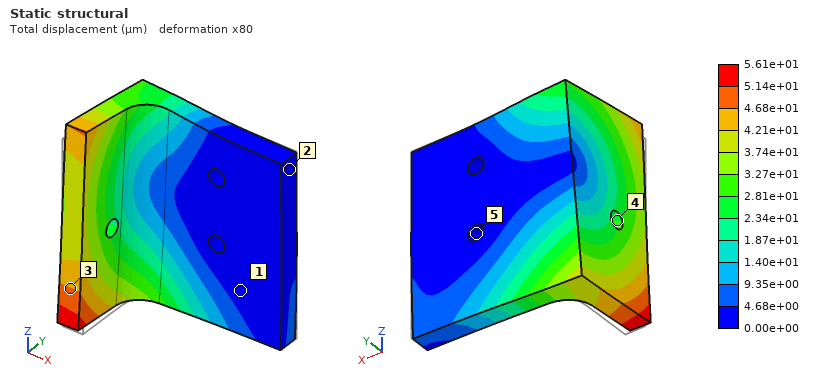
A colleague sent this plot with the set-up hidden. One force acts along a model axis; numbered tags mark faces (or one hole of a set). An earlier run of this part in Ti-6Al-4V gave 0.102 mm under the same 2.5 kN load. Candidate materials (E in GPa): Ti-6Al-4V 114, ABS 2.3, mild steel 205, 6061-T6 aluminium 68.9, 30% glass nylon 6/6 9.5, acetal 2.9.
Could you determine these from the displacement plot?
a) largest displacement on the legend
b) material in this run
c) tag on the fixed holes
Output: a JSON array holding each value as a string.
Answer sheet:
["5.61e+01 µm", "mild steel", "5"]
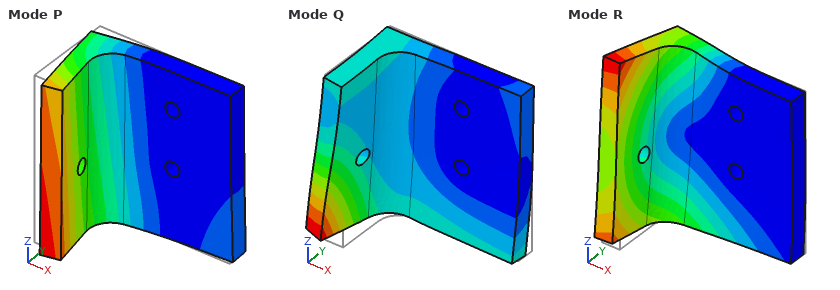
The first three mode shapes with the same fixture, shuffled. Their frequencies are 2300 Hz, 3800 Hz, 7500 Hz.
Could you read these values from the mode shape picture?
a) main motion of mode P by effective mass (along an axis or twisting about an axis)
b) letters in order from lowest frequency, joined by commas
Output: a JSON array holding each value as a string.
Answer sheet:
["along Y", "P, R, Q"]
